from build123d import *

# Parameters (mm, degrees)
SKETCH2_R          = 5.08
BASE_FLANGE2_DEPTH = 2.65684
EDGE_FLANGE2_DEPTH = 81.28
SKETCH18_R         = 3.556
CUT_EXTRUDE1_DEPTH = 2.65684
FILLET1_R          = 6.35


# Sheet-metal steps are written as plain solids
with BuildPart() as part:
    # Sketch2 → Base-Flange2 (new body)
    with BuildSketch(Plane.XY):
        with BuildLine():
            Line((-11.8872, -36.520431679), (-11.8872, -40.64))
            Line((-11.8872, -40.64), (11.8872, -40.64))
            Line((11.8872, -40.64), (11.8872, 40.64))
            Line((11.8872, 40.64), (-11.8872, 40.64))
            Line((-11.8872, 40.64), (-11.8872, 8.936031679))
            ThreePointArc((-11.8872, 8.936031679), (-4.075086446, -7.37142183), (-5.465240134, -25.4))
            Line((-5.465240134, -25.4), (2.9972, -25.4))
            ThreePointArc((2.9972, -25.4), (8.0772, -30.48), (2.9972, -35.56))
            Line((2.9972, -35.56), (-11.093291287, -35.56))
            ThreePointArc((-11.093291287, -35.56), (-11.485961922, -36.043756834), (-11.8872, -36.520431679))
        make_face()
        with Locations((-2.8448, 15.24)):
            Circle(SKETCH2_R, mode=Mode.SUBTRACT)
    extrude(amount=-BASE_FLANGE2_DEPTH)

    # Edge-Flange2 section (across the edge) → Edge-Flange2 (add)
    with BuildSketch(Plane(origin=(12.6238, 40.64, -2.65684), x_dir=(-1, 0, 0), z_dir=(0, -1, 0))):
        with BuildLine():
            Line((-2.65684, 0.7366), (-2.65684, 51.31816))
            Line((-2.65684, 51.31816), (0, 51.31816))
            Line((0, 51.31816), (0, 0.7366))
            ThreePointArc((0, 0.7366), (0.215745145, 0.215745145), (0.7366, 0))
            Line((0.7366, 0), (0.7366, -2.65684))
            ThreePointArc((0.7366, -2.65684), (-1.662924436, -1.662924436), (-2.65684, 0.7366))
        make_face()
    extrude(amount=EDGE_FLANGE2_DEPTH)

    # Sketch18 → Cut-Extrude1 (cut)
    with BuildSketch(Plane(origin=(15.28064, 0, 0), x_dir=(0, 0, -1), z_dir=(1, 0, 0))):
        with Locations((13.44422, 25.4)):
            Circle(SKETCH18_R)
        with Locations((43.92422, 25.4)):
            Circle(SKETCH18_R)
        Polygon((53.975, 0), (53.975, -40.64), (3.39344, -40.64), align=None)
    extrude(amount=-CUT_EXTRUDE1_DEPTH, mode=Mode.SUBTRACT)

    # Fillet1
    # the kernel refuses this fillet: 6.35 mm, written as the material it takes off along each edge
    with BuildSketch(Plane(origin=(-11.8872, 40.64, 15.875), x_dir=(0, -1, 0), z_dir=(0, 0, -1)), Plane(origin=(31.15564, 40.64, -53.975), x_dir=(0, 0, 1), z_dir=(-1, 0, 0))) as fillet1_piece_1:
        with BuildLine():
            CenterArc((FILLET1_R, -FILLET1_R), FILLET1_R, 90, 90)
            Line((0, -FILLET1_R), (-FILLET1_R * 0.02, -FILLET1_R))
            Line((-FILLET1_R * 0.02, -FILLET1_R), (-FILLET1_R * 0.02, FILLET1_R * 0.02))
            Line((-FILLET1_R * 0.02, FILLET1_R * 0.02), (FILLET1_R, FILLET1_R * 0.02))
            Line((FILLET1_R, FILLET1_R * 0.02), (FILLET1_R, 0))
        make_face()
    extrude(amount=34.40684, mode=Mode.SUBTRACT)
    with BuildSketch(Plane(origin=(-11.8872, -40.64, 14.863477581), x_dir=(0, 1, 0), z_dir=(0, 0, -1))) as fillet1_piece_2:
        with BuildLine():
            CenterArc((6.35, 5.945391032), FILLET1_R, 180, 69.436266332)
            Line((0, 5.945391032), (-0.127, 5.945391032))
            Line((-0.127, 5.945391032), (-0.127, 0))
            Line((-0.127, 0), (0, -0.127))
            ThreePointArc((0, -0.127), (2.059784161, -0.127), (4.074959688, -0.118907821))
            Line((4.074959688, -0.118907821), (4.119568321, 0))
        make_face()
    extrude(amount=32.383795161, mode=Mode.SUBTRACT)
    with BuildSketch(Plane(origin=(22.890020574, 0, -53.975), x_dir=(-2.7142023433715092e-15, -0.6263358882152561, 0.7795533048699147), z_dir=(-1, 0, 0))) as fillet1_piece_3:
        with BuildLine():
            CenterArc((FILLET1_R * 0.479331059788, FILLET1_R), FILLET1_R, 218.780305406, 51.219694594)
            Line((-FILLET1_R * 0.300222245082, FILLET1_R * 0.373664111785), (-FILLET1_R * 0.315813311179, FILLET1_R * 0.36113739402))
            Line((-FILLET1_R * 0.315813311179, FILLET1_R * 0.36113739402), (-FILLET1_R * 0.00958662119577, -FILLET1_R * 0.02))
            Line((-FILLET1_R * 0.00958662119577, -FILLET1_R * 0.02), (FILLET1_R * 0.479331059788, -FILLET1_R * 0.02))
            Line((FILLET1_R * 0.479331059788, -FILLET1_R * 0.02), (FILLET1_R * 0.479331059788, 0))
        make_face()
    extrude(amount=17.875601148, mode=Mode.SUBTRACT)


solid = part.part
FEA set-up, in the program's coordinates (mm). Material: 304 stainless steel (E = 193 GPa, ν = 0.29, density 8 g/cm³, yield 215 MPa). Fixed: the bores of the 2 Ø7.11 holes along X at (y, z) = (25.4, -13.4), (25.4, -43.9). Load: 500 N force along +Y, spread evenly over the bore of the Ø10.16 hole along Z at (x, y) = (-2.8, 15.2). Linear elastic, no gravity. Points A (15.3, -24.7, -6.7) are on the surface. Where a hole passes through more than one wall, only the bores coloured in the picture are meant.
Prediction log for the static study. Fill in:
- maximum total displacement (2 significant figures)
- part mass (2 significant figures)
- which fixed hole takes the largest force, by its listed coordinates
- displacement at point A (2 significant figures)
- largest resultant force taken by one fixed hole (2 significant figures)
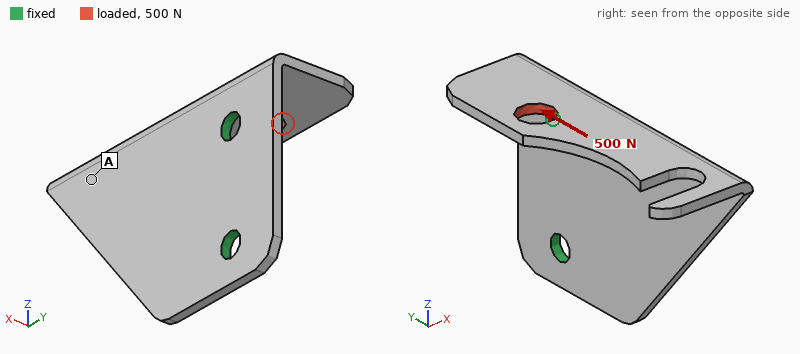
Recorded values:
0.25 mm
99 g
(25.4, -13.4)
0.16 mm
630 N
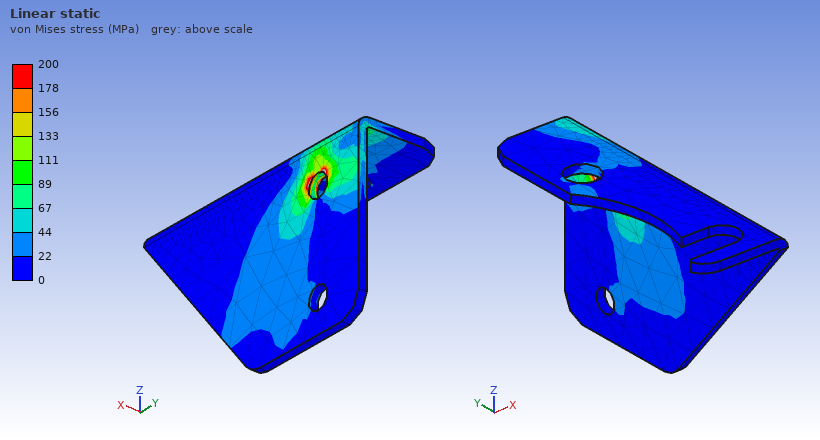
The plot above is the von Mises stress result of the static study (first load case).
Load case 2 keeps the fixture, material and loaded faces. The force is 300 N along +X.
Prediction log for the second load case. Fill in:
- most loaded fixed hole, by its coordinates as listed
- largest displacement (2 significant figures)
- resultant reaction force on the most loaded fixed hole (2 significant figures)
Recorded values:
(25.4, -13.4)
0.10 mm
320 N
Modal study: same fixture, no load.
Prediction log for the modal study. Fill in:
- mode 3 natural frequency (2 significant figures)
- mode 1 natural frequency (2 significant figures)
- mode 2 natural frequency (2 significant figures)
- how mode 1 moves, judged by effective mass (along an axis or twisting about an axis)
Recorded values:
2600 Hz
950 Hz
1800 Hz
along X
